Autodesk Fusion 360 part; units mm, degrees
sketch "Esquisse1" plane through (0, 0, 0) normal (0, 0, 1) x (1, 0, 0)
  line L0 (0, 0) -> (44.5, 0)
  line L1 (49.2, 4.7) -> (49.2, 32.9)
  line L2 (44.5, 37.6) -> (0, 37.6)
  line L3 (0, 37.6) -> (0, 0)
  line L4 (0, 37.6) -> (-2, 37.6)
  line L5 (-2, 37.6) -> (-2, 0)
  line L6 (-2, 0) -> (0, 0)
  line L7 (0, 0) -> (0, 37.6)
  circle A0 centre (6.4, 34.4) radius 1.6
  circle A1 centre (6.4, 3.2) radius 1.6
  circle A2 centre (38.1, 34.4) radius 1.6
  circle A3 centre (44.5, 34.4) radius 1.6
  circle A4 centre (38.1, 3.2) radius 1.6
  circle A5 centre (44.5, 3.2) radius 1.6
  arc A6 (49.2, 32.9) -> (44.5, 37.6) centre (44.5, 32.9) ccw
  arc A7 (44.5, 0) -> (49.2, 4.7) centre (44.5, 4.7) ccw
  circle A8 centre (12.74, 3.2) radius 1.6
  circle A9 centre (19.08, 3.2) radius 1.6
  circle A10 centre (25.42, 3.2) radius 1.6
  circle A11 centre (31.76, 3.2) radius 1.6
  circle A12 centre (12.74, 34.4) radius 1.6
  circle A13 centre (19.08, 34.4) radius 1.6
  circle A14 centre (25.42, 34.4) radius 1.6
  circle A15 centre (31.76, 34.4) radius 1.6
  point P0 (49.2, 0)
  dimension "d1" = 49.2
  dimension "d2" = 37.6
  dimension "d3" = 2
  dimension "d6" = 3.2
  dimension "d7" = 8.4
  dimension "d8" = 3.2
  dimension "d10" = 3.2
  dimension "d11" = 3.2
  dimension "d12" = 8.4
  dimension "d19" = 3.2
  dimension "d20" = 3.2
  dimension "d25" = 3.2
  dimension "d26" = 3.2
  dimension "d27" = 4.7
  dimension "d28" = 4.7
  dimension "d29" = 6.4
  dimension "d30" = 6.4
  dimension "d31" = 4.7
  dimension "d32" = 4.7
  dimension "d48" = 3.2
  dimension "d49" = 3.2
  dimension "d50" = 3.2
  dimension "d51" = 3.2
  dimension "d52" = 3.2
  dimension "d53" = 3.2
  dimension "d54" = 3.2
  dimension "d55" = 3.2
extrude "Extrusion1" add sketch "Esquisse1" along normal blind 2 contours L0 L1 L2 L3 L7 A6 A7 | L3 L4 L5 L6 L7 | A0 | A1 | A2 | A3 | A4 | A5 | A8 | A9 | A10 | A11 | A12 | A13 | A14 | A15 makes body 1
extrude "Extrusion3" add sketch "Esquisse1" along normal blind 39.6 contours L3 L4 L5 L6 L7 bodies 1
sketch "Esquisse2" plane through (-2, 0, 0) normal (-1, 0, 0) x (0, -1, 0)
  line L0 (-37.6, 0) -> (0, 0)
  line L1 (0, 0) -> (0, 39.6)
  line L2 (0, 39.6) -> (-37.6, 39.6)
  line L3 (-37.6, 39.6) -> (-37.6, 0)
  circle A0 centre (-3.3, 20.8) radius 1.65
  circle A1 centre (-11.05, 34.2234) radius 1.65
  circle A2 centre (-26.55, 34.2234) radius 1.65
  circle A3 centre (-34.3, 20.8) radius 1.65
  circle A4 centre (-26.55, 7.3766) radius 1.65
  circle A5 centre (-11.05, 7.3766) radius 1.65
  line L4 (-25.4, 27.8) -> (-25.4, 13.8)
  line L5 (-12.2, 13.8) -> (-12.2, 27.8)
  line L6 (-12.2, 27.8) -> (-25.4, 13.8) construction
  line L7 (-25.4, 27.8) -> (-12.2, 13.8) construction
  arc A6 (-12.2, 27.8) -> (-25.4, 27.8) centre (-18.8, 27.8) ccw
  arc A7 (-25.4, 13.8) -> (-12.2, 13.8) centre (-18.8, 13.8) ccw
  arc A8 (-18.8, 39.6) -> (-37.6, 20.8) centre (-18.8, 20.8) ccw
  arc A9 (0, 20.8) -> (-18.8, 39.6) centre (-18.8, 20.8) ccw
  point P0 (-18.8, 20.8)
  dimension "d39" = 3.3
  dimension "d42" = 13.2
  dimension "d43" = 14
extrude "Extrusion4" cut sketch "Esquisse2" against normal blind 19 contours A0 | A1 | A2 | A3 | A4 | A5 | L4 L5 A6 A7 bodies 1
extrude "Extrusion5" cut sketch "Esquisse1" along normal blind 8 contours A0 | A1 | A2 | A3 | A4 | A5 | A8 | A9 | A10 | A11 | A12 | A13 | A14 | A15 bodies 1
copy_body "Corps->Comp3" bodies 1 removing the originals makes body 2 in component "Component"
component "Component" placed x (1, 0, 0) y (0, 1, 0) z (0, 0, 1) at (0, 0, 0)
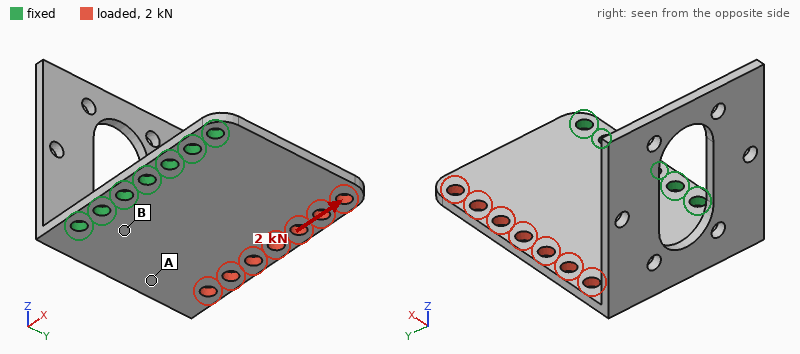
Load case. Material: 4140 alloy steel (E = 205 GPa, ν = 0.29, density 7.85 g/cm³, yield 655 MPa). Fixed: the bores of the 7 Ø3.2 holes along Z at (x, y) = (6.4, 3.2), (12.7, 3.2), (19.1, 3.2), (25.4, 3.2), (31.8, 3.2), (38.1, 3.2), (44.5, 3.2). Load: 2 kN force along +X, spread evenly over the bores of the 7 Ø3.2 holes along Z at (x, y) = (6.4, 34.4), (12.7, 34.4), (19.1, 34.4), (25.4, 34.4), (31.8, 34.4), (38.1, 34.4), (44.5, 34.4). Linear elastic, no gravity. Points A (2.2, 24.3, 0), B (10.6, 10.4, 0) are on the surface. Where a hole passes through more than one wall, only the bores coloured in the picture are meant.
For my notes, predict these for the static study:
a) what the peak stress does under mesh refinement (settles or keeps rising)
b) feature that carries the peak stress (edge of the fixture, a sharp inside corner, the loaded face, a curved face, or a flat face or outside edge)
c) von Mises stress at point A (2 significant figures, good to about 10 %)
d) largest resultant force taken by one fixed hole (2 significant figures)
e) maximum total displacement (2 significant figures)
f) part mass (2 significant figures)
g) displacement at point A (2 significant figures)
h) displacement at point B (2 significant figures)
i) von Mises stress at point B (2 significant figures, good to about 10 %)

keeps rising
edge of the fixture
19 MPa
1.3 kN
18 µm
45 g
11 µm
2.9 µm
57 MPa
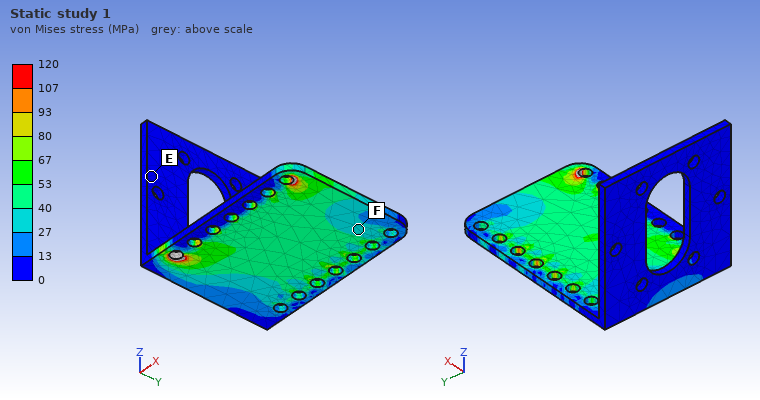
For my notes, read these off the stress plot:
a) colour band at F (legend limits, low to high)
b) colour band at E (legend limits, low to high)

27 to 40 MPa
0 to 13 MPa
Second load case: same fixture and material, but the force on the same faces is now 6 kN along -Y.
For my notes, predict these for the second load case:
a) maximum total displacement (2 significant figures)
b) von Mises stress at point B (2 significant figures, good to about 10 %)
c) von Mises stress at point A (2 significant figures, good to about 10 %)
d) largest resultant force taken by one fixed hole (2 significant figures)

11 µm
63 MPa
31 MPa
1.1 kN
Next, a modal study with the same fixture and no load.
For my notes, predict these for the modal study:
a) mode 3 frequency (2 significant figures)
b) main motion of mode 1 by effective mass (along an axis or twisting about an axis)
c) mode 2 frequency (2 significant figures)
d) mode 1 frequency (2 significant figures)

2000 Hz
along X
1000 Hz
740 Hz
